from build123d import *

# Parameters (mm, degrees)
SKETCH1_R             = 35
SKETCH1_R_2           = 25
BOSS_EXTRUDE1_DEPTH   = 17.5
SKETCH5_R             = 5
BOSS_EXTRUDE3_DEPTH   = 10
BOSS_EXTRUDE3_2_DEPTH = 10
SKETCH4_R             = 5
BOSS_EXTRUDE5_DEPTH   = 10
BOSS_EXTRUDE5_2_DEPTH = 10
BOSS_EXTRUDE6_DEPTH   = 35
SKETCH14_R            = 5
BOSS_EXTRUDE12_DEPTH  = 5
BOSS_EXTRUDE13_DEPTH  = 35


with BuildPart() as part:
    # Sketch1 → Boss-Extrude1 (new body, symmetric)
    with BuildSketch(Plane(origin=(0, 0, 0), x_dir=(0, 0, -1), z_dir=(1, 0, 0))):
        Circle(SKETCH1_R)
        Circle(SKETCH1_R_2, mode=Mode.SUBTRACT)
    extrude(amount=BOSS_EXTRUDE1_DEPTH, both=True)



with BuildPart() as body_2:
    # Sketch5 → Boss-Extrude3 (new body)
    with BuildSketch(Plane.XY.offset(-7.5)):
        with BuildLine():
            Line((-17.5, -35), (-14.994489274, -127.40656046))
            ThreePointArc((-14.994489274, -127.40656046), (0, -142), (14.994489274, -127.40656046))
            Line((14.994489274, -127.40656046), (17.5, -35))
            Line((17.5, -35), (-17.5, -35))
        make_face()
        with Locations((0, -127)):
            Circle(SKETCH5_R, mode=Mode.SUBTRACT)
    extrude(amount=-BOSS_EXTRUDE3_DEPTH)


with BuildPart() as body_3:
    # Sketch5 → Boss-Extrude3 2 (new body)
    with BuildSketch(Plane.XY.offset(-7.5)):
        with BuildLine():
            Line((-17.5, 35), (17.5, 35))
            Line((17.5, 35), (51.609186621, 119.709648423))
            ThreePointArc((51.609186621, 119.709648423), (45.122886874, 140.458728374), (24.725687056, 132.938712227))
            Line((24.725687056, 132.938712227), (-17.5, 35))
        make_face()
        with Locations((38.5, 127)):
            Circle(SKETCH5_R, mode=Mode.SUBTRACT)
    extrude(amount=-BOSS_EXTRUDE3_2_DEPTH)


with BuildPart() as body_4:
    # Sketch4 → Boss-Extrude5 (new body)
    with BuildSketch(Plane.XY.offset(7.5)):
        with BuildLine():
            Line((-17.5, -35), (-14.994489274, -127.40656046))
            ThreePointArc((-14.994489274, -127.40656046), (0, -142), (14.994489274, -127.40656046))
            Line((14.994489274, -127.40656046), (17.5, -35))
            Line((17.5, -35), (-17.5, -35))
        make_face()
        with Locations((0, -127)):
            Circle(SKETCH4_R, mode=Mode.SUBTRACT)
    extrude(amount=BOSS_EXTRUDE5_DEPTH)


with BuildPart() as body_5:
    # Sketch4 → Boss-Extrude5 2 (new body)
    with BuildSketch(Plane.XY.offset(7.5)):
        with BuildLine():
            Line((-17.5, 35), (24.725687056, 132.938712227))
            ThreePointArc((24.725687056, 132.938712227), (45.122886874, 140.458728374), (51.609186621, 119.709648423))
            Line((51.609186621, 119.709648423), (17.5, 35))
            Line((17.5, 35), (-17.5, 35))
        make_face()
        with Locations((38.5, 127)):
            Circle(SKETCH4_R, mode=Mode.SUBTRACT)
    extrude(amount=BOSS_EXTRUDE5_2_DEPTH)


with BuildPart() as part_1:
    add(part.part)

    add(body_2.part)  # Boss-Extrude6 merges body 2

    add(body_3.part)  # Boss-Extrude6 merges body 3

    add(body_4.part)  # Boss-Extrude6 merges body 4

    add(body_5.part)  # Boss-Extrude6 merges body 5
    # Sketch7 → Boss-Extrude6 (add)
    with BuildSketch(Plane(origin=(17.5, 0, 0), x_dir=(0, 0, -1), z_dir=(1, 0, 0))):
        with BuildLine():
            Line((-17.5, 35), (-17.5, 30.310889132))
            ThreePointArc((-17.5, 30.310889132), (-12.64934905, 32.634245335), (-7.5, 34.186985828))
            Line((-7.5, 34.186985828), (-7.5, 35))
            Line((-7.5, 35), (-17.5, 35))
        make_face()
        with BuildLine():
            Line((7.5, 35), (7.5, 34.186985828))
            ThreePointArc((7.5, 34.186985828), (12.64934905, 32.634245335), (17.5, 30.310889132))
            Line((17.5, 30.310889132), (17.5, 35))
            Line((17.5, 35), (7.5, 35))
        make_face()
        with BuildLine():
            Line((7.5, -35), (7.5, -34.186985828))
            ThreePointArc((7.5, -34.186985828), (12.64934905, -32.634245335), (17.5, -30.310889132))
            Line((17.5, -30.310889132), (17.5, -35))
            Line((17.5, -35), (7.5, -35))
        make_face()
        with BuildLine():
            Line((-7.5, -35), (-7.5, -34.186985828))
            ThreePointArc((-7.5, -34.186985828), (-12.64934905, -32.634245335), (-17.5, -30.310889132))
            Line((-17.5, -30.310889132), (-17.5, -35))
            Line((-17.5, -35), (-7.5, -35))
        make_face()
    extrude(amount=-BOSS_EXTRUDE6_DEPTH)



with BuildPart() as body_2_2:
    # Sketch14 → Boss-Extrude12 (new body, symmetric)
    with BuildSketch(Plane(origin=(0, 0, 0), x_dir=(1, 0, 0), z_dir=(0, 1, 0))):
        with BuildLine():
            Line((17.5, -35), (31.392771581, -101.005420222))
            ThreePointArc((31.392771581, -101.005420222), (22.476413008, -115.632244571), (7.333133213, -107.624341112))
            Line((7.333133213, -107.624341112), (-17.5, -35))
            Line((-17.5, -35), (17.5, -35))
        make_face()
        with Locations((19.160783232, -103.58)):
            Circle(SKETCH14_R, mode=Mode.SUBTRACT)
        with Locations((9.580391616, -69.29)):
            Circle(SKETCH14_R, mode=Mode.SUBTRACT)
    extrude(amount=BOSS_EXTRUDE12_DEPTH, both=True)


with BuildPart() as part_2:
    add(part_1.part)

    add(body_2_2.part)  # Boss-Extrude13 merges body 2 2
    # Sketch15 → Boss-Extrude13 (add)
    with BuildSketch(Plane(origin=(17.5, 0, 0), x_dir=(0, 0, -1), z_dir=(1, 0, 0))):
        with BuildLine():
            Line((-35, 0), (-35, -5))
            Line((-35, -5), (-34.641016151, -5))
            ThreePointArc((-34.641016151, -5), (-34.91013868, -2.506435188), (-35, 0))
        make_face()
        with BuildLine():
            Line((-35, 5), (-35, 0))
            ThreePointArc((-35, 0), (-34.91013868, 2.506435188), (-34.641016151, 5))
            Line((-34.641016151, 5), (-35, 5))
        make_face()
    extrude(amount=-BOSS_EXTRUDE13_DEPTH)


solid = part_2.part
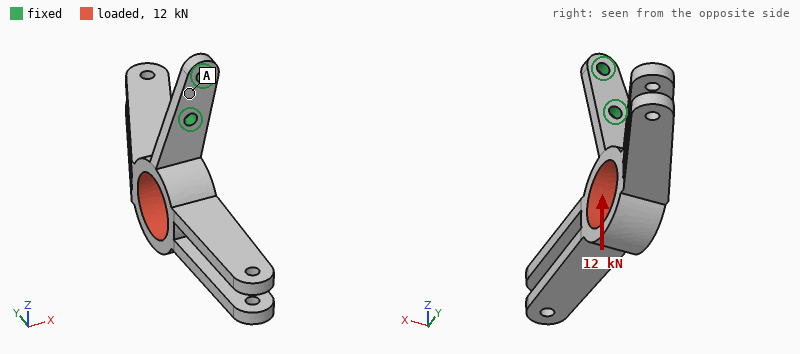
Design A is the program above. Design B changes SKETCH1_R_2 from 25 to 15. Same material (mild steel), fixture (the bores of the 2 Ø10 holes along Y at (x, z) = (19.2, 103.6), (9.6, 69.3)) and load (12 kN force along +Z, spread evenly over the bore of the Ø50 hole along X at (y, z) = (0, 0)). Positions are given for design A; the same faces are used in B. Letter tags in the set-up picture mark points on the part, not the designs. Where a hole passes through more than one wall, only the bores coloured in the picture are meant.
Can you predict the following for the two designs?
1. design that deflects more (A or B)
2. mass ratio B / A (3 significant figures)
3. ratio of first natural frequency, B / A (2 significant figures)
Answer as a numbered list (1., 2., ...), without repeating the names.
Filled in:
1. A
2. 1.20
3. 1.0
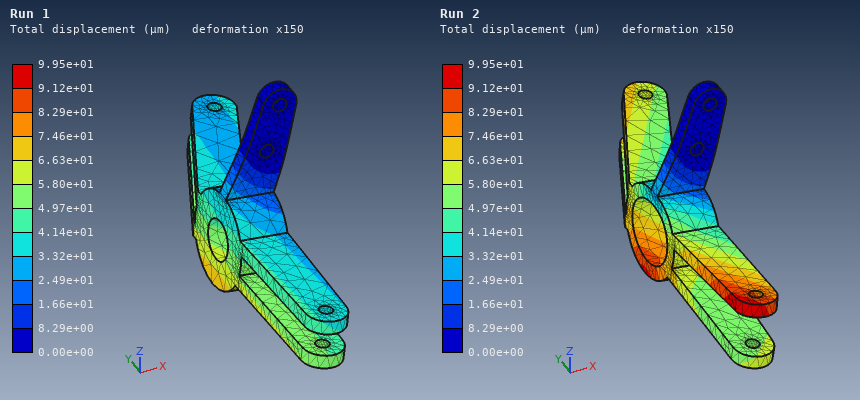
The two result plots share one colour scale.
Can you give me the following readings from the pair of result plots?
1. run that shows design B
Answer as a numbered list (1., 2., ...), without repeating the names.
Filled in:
1. Run 1
